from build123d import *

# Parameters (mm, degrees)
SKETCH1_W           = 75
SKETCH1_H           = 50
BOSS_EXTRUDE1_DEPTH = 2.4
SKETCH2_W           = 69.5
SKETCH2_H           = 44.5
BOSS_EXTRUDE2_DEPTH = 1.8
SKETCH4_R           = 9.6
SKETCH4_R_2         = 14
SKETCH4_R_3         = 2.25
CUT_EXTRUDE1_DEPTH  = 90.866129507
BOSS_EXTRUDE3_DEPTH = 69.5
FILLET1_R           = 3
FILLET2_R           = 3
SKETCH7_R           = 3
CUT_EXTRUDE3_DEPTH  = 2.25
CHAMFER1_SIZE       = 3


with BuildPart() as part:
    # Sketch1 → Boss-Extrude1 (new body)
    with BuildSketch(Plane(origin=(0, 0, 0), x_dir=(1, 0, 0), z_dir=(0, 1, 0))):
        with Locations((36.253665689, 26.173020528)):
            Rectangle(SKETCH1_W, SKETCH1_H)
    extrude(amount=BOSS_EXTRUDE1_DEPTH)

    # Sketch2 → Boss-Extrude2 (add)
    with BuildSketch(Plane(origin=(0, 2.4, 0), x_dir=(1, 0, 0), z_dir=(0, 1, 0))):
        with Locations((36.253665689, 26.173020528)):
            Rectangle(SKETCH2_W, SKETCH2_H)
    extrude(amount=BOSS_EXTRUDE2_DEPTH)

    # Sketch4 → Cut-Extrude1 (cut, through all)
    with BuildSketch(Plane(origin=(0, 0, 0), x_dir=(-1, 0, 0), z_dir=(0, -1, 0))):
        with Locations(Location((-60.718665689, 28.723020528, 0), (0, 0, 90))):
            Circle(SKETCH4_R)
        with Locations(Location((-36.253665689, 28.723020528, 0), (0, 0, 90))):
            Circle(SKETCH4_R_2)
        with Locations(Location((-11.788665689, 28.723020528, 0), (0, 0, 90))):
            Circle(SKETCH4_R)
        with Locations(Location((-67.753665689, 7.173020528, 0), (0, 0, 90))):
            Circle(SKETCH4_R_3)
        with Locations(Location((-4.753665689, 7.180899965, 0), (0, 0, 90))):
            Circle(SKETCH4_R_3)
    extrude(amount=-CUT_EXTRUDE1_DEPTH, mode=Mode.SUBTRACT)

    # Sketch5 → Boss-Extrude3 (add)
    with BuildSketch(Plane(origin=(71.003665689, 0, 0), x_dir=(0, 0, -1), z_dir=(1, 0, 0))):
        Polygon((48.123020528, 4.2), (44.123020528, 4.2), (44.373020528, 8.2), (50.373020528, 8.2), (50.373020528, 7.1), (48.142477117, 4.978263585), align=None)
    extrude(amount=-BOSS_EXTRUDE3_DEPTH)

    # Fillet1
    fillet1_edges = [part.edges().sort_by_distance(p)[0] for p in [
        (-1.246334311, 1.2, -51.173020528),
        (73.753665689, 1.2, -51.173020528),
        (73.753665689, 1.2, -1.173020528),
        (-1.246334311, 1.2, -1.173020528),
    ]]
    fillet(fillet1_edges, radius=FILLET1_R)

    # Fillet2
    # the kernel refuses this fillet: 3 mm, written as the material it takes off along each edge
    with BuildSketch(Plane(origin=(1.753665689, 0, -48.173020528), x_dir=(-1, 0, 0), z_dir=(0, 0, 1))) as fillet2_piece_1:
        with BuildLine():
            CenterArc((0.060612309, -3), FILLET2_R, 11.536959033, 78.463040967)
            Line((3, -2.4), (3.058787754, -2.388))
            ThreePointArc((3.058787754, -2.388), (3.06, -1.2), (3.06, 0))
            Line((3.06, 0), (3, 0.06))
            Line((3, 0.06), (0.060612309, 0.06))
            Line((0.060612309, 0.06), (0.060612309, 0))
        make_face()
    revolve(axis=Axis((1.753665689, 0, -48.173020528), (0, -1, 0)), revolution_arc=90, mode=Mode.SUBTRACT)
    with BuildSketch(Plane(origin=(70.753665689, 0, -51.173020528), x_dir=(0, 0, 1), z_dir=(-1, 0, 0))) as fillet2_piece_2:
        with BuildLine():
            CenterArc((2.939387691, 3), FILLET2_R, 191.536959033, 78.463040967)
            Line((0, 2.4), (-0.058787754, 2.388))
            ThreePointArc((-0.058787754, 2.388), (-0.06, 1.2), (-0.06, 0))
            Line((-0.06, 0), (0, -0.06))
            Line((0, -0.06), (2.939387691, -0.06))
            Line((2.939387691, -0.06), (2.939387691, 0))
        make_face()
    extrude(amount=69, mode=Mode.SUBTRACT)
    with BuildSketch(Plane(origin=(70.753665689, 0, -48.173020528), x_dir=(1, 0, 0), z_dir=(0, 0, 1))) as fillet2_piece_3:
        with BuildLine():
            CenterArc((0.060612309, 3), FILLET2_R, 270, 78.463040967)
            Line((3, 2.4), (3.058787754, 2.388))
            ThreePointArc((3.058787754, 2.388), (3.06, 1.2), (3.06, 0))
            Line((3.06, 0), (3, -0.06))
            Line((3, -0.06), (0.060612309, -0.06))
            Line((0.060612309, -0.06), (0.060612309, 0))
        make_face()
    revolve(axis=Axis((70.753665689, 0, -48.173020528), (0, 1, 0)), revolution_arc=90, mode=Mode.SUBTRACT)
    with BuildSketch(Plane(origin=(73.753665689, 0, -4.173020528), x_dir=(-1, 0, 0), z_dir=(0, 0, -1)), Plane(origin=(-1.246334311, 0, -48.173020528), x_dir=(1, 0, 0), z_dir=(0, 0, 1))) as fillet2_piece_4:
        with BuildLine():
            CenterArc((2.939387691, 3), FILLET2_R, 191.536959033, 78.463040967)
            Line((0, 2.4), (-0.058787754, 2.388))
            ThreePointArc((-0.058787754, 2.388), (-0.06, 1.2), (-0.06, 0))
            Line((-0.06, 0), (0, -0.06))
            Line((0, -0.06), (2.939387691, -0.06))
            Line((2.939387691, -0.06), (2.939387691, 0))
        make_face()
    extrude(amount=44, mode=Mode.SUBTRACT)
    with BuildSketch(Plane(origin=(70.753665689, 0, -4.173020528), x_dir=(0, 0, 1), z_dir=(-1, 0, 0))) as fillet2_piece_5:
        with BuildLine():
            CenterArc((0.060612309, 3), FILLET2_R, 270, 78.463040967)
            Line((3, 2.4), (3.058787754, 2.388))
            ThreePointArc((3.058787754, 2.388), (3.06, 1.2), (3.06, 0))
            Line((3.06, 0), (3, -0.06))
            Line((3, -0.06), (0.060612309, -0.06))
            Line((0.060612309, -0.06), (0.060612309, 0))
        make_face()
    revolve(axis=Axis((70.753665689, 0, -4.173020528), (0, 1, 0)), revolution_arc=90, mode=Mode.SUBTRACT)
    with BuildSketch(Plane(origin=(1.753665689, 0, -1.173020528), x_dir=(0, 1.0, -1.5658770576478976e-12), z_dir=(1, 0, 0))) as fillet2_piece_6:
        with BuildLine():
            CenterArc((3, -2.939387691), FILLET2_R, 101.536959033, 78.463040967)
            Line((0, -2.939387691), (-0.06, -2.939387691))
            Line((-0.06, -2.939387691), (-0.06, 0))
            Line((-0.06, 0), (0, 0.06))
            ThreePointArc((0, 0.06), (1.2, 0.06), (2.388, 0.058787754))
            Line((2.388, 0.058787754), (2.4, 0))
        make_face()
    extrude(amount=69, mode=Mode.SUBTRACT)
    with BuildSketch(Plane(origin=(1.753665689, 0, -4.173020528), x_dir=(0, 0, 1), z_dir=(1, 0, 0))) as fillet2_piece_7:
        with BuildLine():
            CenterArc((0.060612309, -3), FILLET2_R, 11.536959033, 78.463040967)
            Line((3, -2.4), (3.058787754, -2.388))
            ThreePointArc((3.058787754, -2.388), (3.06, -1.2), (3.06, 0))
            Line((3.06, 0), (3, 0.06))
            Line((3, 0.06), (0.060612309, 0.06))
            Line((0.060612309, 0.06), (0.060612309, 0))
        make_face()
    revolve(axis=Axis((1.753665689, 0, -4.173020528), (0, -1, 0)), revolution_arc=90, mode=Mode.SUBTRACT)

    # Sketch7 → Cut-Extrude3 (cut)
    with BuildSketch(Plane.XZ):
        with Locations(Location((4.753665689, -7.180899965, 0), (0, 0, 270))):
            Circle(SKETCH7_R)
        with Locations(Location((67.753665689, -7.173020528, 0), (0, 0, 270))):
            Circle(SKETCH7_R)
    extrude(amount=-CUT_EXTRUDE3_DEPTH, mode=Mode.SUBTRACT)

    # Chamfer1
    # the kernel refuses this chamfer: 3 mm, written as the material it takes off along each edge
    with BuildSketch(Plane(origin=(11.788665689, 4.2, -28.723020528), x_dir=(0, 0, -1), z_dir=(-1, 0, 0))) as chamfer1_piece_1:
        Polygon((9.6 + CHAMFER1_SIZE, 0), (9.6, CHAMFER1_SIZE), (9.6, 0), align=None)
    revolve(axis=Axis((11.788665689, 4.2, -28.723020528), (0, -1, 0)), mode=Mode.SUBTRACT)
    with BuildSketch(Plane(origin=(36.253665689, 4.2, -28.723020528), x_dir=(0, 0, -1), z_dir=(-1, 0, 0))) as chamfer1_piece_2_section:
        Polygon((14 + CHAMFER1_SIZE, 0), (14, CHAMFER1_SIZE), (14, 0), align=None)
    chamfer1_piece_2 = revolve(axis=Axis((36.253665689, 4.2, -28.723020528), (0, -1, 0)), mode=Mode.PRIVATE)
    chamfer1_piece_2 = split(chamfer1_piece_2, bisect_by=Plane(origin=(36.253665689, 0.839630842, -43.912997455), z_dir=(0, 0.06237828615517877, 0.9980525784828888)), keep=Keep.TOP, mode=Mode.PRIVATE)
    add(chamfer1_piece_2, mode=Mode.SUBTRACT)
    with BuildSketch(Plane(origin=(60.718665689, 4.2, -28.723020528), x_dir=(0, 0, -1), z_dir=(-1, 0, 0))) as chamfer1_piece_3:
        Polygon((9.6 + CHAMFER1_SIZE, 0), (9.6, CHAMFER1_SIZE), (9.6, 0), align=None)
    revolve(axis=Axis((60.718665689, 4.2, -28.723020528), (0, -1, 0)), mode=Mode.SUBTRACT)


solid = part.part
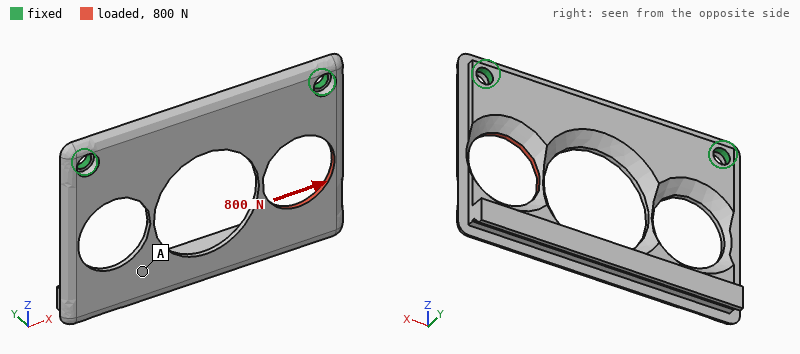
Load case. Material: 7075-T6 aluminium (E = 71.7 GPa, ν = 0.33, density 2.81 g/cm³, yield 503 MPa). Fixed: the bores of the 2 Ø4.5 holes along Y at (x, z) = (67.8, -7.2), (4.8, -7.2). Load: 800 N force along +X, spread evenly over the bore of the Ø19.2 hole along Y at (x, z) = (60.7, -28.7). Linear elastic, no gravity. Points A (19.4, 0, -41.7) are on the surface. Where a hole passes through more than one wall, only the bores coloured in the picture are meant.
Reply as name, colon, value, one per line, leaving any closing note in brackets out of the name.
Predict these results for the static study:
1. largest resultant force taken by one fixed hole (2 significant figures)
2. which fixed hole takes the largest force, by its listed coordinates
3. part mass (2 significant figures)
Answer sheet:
largest resultant force taken by one fixed hole: 520 N
which fixed hole takes the largest force, by its listed coordinates: (67.8, -7.2)
part mass: 27 g
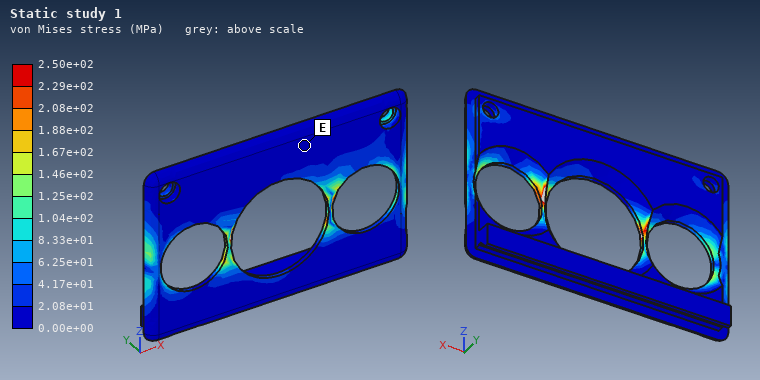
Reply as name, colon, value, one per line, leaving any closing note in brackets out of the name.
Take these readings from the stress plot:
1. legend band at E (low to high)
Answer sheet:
legend band at E: 0.00e+00 to 2.08e+01 MPa
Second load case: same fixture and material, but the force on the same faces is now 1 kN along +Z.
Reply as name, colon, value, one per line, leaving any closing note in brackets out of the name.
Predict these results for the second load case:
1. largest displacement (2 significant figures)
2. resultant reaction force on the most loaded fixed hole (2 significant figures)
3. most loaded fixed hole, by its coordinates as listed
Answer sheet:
largest displacement: 0.31 mm
resultant reaction force on the most loaded fixed hole: 890 N
most loaded fixed hole, by its coordinates as listed: (67.8, -7.2)
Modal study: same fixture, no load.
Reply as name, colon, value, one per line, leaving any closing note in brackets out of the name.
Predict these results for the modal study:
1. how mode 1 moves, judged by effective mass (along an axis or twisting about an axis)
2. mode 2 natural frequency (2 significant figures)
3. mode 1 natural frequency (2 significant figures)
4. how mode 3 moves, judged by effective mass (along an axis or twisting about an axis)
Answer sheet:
how mode 1 moves, judged by effective mass: along Y
mode 2 natural frequency: 1700 Hz
mode 1 natural frequency: 450 Hz
how mode 3 moves, judged by effective mass: along X
